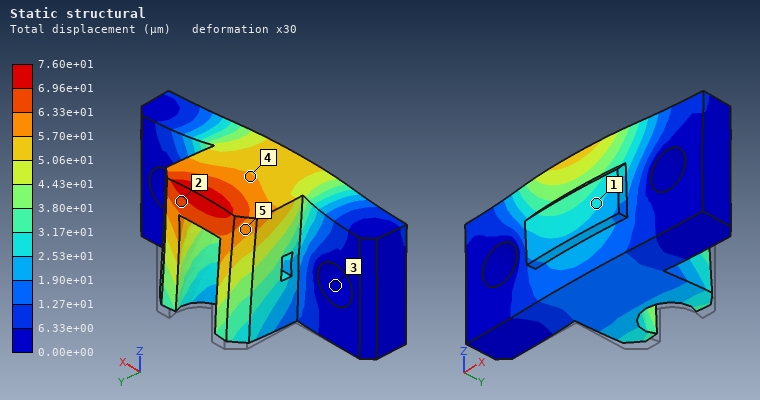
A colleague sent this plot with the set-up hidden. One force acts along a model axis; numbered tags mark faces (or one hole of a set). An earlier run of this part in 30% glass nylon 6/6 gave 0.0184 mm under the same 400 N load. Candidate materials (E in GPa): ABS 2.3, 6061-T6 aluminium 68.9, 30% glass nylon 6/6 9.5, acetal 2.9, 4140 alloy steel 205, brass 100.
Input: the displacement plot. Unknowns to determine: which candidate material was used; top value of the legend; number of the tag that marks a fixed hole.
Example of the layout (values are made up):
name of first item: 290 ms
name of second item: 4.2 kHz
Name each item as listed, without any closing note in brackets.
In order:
which candidate material was used: ABS
top value of the legend: 7.60e+01 µm
number of the tag that marks a fixed hole: 3
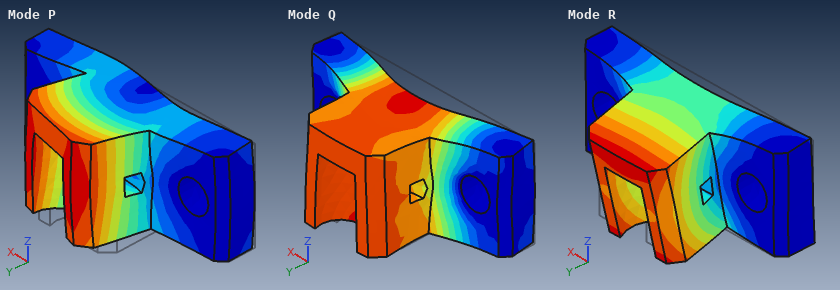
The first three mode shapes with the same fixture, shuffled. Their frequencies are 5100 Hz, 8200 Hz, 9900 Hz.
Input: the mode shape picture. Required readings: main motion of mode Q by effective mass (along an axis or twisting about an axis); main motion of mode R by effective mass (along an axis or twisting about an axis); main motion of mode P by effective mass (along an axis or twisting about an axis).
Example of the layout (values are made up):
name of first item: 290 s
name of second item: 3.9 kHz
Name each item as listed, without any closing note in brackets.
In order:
main motion of mode Q by effective mass: along Y
main motion of mode R by effective mass: along Z
main motion of mode P by effective mass: along X
